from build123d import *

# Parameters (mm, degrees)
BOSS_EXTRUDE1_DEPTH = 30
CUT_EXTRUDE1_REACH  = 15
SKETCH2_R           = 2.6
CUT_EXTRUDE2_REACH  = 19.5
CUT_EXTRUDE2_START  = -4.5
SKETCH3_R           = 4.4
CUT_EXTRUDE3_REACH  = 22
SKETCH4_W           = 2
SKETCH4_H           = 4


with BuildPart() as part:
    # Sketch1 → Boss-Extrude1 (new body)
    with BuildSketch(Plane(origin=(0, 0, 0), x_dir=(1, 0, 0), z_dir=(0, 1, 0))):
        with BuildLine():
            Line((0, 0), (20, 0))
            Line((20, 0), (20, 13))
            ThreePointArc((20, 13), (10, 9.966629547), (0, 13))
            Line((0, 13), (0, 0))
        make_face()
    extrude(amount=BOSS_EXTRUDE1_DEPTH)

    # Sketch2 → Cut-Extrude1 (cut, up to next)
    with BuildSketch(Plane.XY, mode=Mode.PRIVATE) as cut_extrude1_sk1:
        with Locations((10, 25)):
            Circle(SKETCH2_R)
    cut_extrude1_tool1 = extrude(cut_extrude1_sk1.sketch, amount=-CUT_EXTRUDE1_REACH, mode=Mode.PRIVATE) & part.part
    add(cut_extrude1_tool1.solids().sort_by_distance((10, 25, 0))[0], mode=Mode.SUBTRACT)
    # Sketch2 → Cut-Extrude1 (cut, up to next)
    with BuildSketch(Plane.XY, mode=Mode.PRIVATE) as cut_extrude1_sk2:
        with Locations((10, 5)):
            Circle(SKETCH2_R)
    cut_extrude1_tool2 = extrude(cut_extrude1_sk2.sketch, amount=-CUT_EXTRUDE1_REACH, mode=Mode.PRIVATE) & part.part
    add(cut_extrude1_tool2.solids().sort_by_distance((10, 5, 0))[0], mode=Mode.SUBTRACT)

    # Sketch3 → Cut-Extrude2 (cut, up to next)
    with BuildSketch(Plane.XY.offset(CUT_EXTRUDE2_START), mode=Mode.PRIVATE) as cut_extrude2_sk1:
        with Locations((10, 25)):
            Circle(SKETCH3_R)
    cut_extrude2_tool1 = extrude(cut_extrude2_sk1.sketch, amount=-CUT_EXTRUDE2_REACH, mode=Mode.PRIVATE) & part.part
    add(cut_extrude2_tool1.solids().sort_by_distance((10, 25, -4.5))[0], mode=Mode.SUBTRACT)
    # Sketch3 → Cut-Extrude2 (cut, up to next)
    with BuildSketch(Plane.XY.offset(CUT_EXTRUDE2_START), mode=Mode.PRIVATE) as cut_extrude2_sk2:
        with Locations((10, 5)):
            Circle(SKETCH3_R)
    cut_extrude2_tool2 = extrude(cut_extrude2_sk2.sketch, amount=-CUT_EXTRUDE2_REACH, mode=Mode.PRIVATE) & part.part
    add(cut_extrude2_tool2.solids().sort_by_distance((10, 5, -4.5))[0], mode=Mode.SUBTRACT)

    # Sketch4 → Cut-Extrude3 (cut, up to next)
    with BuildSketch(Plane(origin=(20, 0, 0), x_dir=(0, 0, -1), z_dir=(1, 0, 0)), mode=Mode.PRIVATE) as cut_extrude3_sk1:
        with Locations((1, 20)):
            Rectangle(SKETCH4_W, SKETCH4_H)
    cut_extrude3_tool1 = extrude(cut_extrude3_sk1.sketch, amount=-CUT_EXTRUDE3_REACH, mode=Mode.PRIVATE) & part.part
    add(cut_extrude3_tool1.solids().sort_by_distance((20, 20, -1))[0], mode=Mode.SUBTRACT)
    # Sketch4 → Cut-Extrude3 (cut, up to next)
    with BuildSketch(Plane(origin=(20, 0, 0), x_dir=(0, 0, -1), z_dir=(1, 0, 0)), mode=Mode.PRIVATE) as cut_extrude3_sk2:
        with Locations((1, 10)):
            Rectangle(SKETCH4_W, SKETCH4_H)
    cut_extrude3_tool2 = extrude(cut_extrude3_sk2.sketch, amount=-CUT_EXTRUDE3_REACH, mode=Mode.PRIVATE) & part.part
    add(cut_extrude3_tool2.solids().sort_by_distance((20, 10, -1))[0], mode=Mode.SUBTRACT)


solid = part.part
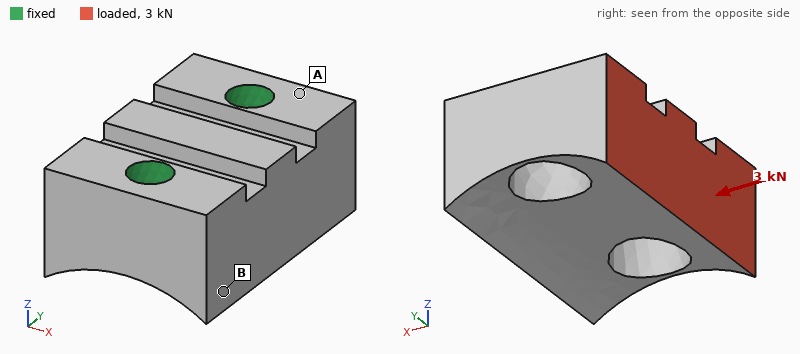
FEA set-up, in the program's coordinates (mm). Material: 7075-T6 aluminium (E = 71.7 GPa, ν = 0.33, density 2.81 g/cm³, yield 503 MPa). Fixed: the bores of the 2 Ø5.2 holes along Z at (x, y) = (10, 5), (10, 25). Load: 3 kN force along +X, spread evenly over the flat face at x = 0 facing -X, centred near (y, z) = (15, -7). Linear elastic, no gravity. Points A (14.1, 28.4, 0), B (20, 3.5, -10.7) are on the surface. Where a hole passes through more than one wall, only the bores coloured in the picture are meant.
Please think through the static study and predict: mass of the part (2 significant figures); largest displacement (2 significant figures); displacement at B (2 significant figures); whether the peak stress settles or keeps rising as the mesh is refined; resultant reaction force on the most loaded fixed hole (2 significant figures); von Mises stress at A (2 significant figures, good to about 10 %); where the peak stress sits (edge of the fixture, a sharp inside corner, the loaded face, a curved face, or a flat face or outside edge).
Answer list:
15 g
25 µm
13 µm
keeps rising
1.5 kN
22 MPa
edge of the fixture
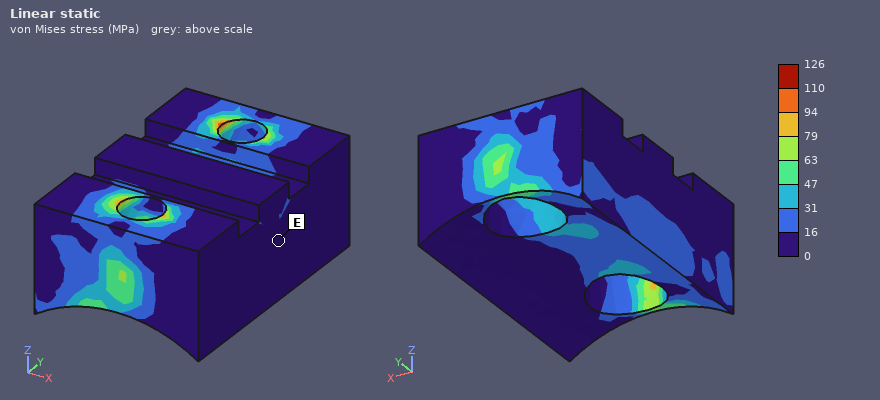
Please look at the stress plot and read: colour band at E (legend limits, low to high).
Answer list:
0 to 16 MPa
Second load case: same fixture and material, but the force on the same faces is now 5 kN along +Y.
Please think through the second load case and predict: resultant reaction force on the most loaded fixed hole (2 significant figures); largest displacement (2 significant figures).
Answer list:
3.3 kN
23 µm
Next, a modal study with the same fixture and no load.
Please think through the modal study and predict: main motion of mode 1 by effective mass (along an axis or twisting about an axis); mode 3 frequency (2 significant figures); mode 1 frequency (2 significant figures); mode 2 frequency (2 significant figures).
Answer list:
along X
35 kHz
18 kHz
34 kHz
